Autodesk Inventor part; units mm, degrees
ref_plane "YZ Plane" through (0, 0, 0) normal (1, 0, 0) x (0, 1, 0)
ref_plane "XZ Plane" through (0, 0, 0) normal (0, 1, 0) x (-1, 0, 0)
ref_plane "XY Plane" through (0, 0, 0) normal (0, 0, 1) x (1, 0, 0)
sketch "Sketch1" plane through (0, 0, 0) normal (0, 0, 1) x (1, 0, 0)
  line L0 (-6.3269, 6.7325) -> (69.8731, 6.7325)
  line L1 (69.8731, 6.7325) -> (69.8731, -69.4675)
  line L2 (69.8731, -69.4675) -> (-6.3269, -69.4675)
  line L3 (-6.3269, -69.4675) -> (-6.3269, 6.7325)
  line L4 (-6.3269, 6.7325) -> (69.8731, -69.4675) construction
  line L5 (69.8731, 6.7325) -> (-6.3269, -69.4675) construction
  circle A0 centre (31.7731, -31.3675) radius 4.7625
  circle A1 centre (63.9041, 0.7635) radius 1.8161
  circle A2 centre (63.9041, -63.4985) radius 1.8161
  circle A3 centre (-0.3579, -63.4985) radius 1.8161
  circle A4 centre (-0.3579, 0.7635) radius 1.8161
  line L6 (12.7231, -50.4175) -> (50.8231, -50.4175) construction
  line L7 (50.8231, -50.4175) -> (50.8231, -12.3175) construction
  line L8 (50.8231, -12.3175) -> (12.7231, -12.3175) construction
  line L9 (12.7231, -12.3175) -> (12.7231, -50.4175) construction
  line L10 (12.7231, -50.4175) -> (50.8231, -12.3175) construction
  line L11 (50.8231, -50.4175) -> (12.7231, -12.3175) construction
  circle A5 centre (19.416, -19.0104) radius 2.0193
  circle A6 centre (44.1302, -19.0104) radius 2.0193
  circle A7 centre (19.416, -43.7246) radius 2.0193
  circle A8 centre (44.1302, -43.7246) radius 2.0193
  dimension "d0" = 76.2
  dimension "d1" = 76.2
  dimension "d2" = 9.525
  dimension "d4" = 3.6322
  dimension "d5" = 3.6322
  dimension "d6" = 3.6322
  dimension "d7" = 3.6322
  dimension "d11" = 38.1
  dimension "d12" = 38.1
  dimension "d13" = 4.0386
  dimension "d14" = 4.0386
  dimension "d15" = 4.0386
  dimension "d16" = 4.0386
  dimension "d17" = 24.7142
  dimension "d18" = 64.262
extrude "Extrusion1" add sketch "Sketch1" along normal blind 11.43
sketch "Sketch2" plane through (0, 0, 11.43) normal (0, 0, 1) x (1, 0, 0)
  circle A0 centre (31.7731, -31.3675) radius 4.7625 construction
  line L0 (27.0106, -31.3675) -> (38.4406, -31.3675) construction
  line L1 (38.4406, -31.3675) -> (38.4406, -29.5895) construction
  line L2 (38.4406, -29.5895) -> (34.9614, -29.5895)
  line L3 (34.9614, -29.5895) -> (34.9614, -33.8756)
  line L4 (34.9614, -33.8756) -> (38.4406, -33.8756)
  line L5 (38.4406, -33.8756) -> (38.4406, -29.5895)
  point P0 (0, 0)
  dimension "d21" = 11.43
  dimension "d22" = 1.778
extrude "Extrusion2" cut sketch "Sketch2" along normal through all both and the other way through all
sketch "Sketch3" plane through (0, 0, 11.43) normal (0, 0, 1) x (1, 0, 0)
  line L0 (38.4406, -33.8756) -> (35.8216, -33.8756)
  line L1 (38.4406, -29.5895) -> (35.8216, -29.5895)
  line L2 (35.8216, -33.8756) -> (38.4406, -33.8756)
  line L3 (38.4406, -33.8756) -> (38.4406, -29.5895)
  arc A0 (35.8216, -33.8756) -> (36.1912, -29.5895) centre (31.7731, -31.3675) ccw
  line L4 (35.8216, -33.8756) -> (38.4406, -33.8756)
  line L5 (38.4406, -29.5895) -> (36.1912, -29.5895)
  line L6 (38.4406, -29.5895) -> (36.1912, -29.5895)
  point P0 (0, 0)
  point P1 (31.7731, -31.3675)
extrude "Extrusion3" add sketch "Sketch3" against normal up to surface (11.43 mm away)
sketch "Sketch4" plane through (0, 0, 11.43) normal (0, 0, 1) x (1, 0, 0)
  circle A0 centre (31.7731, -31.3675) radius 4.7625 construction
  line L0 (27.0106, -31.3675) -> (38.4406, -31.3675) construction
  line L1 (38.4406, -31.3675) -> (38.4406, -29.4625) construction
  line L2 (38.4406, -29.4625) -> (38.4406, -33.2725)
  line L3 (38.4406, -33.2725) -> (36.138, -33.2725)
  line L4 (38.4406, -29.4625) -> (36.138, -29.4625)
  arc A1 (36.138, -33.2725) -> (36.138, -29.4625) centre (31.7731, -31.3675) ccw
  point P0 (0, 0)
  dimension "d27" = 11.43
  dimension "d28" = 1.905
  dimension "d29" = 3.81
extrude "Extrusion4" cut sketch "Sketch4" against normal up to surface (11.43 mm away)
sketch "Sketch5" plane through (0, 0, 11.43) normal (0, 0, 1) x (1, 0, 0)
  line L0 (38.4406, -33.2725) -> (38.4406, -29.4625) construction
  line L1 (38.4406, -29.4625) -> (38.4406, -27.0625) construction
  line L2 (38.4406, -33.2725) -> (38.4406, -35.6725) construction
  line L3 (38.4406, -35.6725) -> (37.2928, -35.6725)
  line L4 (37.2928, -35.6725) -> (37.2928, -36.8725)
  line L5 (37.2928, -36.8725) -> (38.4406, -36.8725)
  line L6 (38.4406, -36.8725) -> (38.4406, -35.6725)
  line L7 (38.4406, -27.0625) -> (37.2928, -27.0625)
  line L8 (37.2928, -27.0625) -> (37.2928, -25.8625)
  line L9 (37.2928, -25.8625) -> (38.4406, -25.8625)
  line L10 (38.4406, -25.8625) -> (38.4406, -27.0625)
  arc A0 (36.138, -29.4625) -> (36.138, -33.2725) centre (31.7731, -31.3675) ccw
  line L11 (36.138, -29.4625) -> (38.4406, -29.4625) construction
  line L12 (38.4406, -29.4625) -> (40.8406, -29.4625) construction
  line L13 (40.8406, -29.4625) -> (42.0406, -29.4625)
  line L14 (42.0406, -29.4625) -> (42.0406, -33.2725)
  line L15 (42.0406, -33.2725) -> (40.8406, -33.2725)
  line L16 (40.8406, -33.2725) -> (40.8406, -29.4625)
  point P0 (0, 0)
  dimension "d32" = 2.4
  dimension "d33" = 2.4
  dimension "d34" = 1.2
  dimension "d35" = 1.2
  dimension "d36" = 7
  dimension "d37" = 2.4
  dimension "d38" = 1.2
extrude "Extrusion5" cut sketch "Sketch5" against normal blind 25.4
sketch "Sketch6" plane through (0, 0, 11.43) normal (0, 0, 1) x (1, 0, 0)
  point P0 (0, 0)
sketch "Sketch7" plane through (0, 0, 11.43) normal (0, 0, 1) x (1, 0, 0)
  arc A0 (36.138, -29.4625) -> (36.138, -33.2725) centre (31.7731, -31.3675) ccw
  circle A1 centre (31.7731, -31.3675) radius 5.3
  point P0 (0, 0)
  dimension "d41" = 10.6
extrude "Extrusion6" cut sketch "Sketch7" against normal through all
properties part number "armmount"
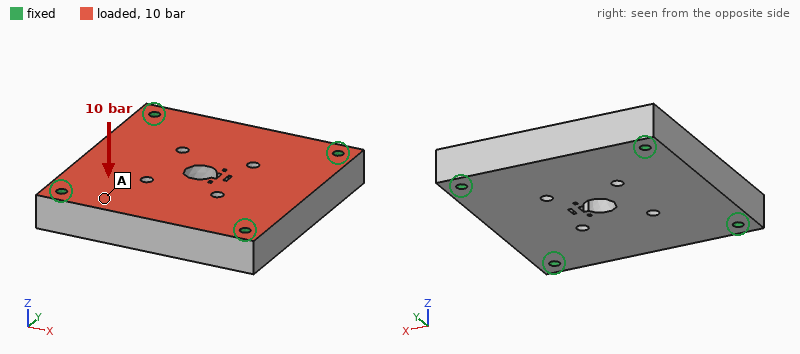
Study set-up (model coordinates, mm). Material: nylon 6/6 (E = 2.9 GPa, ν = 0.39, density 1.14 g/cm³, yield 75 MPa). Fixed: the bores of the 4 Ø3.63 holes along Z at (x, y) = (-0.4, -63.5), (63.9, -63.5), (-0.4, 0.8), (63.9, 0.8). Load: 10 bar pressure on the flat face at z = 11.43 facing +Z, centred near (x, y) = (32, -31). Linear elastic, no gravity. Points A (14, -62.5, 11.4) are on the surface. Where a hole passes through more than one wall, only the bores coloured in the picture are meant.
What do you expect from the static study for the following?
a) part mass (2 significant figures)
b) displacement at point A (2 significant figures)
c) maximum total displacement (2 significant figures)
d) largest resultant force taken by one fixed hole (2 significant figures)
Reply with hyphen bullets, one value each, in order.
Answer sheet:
- 73 g
- 0.20 mm
- 0.52 mm
- 1.4 kN
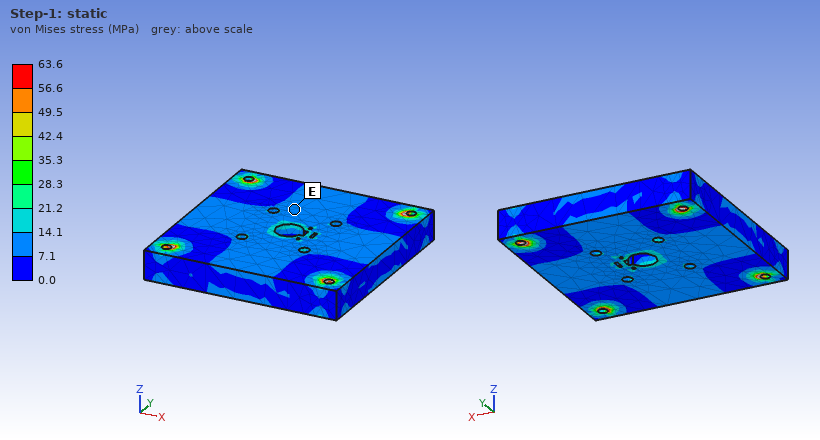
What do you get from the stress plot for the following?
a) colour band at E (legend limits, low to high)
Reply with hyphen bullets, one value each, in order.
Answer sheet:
- 7.1 to 14.1 MPa
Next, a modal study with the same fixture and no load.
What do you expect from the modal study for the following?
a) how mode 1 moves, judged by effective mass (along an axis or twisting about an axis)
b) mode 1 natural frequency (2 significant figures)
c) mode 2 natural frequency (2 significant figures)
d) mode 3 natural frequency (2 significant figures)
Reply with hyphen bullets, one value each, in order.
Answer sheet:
- along Z
- 2400 Hz
- 3800 Hz
- 3800 Hz
